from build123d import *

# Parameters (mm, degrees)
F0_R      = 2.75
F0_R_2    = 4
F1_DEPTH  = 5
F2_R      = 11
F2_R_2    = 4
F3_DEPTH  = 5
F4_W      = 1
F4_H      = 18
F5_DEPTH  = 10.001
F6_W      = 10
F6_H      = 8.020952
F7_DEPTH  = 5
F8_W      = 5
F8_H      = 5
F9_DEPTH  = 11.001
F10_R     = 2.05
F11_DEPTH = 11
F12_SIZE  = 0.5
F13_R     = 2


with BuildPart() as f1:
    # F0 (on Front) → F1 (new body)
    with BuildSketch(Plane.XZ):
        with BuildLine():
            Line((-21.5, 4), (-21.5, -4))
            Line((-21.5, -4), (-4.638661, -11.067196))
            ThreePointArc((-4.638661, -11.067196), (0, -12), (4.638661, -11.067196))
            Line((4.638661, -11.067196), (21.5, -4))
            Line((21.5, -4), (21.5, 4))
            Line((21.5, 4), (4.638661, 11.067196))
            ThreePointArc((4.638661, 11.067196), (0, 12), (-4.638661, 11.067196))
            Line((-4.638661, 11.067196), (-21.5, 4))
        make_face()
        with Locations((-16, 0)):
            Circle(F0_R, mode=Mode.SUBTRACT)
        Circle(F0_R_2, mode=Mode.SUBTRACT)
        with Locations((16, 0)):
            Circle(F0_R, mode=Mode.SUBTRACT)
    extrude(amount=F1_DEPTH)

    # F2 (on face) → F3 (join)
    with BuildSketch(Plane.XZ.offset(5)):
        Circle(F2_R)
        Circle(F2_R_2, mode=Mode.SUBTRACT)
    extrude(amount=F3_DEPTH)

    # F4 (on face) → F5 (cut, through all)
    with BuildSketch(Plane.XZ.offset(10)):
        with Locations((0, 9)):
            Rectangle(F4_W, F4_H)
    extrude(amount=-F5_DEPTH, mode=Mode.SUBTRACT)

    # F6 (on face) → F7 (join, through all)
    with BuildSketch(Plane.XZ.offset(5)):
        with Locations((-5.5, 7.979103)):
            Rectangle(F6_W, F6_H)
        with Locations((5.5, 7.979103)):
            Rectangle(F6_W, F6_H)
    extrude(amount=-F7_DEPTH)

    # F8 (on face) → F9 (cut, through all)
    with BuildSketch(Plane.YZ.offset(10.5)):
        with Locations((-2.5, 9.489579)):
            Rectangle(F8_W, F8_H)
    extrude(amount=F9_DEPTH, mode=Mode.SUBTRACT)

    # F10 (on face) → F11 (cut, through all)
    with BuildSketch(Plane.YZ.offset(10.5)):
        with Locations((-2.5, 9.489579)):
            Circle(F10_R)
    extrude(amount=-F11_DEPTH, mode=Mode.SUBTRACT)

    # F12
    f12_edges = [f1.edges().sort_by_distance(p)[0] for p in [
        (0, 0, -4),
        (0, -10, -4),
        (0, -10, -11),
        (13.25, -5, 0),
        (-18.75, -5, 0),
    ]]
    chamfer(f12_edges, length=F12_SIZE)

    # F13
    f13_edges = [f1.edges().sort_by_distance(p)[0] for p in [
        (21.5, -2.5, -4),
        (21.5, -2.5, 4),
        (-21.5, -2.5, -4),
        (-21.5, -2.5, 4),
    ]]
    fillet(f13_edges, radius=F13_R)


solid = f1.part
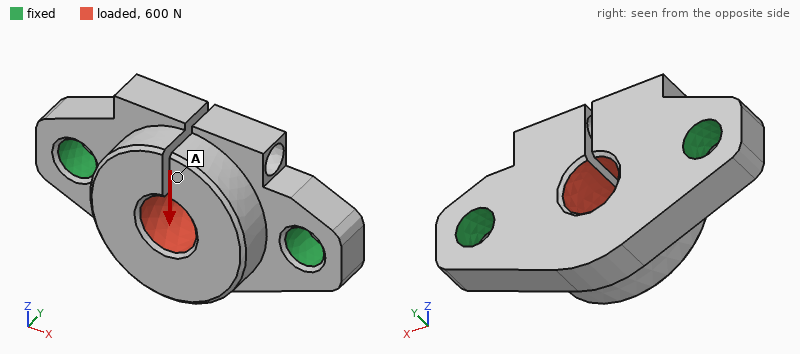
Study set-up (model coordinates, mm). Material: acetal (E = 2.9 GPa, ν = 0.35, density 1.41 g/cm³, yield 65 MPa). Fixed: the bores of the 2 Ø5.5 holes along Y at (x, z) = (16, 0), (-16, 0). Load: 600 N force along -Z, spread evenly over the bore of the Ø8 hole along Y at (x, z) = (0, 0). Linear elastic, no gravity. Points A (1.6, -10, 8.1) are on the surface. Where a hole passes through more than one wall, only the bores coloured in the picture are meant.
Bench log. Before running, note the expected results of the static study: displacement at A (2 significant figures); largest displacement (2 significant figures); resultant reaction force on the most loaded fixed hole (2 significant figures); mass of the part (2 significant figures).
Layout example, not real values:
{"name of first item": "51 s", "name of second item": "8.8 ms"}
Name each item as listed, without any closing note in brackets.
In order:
{"displacement at A": "0.16 mm", "largest displacement": "0.17 mm", "resultant reaction force on the most loaded fixed hole": "390 N", "mass of the part": "6.6 g"}
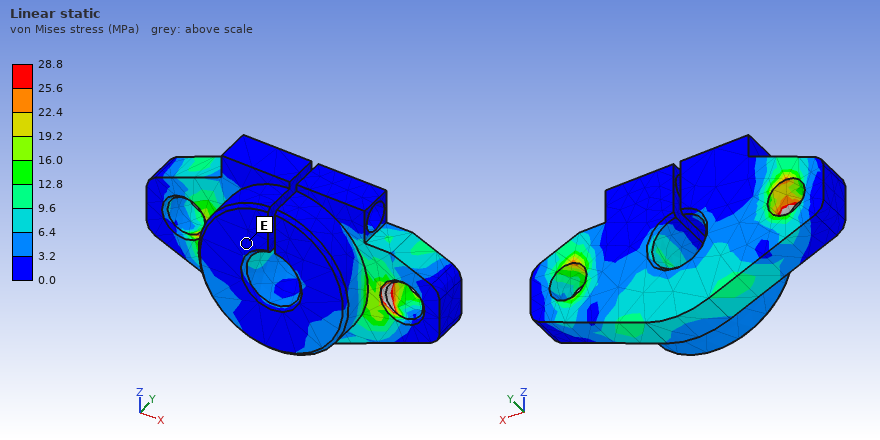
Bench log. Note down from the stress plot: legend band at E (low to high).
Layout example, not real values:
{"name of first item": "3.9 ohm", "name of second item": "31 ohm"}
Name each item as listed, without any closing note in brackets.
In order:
{"legend band at E": "0.0 to 3.2 MPa"}
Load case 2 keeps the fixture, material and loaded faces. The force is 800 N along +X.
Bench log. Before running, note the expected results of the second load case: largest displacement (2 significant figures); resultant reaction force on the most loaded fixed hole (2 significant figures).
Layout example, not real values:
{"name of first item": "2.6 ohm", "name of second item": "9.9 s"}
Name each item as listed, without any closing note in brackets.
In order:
{"largest displacement": "80 µm", "resultant reaction force on the most loaded fixed hole": "400 N"}
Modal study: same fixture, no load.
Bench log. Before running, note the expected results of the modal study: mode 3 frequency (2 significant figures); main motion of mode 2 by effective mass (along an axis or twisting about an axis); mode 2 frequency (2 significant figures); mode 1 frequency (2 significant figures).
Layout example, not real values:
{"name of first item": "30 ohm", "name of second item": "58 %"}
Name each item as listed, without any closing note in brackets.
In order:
{"mode 3 frequency": "5300 Hz", "main motion of mode 2 by effective mass": "along Y", "mode 2 frequency": "5000 Hz", "mode 1 frequency": "4400 Hz"}
